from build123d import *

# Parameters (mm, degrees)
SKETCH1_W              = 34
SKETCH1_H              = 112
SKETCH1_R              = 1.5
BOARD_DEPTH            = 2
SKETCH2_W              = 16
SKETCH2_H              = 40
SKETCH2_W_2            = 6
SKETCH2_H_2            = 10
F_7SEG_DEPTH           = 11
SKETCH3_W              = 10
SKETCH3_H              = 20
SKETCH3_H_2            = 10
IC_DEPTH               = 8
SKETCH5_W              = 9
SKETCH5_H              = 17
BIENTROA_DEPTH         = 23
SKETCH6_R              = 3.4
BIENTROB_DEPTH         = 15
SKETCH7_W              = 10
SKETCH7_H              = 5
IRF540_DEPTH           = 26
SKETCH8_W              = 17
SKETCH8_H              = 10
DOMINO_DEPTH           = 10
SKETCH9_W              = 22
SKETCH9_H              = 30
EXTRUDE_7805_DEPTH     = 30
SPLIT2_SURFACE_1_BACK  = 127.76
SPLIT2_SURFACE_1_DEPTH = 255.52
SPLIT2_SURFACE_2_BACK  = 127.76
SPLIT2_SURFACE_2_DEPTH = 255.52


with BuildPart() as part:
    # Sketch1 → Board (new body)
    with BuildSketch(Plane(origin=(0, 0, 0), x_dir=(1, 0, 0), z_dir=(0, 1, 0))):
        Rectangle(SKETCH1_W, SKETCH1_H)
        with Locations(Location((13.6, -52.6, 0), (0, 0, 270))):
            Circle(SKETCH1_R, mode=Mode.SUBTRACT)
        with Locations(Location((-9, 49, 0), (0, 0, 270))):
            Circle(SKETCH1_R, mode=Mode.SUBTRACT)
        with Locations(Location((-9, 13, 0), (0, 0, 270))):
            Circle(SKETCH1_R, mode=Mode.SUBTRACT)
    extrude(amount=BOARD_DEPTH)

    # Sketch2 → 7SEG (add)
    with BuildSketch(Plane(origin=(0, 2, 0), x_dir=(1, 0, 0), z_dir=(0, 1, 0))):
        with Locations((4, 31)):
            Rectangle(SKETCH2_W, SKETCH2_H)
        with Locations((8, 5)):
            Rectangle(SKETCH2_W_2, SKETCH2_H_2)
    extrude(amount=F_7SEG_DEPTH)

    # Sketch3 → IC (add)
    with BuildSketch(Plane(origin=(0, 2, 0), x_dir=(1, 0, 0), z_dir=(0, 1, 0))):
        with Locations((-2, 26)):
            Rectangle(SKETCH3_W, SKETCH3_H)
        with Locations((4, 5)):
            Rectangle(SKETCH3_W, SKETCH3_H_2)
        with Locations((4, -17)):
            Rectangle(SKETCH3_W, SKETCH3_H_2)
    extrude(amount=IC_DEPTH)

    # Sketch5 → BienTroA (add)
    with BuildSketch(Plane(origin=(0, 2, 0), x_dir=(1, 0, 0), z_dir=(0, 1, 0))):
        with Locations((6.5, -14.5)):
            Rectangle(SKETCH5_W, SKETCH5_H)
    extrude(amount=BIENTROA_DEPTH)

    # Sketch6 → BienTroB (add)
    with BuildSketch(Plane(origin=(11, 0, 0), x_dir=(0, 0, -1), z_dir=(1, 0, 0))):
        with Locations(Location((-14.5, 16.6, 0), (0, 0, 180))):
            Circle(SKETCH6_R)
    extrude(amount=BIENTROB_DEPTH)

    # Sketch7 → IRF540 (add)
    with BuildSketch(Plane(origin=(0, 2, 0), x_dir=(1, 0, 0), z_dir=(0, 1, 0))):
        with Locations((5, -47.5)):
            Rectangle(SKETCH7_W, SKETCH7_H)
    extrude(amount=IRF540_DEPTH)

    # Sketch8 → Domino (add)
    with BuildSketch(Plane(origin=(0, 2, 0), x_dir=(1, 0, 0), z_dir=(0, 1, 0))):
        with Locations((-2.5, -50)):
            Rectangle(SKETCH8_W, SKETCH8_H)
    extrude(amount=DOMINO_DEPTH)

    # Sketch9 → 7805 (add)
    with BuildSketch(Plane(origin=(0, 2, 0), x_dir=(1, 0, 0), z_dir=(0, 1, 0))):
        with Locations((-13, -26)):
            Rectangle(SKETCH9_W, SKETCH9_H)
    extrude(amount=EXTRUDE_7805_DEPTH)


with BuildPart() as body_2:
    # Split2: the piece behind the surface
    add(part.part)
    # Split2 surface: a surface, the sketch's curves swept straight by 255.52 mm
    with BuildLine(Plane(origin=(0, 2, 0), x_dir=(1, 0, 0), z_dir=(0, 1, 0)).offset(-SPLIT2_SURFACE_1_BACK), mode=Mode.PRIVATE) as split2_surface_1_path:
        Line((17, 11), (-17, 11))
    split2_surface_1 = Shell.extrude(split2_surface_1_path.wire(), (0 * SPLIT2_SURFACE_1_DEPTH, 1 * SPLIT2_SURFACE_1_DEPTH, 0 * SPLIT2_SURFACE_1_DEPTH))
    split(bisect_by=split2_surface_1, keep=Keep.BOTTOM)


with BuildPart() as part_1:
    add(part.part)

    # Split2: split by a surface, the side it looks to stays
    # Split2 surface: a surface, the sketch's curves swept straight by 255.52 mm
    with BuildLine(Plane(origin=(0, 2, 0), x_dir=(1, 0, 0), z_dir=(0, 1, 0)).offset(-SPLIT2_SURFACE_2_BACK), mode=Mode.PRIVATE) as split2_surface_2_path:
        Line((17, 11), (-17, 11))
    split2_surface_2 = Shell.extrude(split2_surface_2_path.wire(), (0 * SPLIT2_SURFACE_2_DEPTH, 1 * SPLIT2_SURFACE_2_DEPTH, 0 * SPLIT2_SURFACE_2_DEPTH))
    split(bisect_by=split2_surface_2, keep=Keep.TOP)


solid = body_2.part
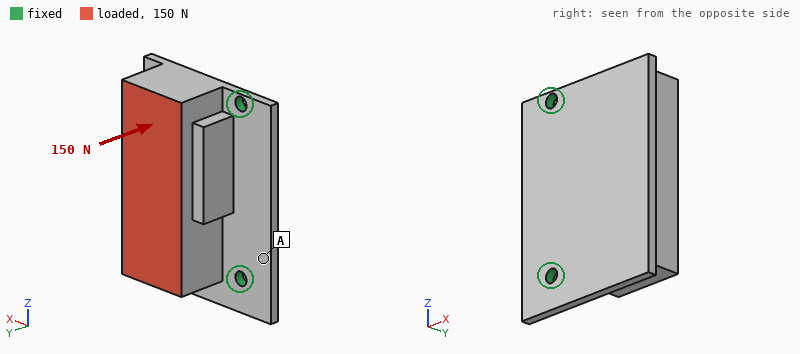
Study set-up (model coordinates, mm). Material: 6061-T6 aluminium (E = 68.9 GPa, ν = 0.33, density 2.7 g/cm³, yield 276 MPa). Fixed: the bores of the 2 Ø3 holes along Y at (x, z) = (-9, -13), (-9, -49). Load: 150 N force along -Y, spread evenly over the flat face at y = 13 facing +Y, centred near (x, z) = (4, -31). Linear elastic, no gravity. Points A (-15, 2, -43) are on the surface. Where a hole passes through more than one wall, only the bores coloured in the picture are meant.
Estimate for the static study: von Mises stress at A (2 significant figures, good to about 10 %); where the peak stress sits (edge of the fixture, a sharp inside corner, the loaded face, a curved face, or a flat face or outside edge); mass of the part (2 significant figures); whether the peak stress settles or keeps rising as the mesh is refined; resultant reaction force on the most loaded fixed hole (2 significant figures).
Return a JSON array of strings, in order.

["14 MPa", "edge of the fixture", "28 g", "keeps rising", "77 N"]
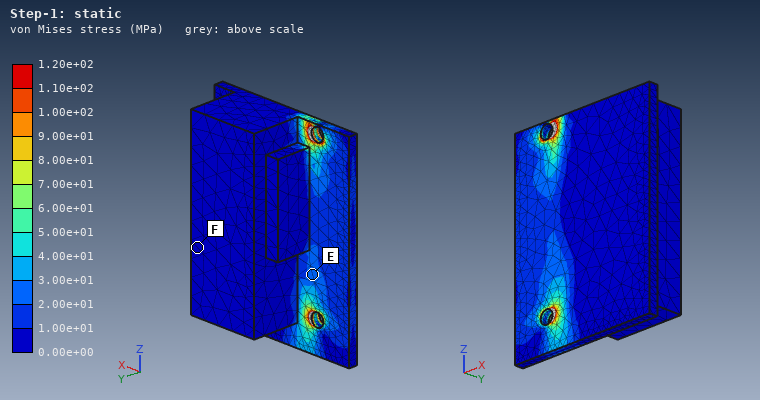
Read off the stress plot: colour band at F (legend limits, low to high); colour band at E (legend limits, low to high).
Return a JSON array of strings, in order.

["0.00e+00 to 1.00e+01 MPa", "2.00e+01 to 3.00e+01 MPa"]
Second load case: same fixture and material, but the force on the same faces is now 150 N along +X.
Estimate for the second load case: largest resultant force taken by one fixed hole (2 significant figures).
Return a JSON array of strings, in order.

["78 N"]
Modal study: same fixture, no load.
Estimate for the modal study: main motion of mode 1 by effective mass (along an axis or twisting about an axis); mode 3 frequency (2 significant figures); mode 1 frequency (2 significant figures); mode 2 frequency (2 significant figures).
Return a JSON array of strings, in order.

["along Y", "11 kHz", "1300 Hz", "8300 Hz"]
